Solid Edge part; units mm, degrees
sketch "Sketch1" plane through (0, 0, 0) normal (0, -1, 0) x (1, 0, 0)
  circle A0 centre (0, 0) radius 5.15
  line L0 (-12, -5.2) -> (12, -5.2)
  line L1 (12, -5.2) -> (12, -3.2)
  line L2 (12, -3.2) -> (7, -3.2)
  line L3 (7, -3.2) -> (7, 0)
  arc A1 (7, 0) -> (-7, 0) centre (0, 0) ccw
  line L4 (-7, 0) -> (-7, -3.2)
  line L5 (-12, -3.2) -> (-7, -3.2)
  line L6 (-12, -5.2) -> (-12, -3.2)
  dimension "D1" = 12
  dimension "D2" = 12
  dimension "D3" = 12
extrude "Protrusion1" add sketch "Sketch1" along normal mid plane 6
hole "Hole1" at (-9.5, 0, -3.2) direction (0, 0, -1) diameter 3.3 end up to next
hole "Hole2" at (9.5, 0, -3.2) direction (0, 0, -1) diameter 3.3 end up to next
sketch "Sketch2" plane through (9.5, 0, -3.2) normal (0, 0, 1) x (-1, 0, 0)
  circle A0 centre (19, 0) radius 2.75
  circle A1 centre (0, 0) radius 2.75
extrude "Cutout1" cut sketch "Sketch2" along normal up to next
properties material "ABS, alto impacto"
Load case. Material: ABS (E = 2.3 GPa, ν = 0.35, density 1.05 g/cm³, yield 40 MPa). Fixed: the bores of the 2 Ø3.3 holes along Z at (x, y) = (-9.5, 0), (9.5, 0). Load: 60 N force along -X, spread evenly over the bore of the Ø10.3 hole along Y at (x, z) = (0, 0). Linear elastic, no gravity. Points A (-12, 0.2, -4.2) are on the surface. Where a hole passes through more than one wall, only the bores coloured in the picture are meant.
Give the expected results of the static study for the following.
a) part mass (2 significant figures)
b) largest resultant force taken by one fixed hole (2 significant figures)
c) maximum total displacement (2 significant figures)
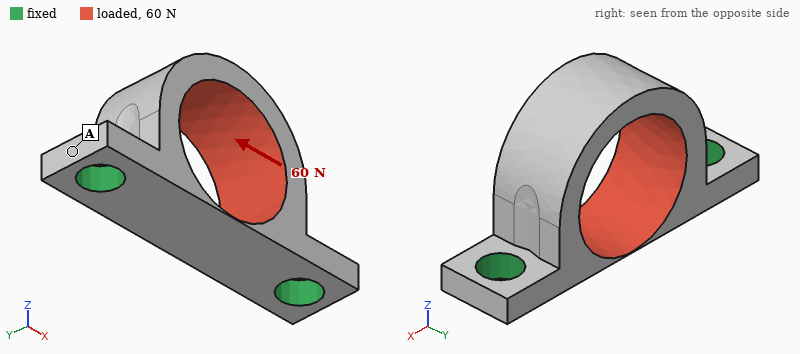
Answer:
0.51 g
32 N
0.14 mm
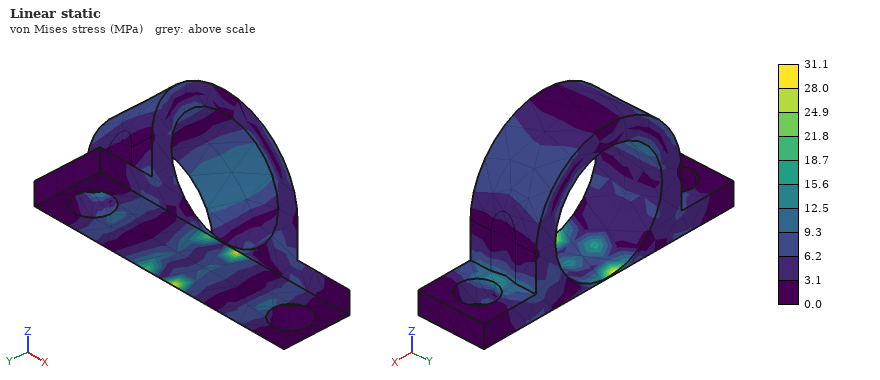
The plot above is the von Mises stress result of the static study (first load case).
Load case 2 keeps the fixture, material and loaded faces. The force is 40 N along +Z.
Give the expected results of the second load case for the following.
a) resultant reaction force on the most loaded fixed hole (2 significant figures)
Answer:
20 N
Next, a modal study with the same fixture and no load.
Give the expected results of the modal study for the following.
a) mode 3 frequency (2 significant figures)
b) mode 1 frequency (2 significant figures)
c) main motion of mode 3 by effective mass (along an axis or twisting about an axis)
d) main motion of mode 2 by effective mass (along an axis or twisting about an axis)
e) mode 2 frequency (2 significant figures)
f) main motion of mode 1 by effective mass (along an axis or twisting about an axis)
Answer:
9100 Hz
4400 Hz
twisting about Z
along X
5400 Hz
along Y
